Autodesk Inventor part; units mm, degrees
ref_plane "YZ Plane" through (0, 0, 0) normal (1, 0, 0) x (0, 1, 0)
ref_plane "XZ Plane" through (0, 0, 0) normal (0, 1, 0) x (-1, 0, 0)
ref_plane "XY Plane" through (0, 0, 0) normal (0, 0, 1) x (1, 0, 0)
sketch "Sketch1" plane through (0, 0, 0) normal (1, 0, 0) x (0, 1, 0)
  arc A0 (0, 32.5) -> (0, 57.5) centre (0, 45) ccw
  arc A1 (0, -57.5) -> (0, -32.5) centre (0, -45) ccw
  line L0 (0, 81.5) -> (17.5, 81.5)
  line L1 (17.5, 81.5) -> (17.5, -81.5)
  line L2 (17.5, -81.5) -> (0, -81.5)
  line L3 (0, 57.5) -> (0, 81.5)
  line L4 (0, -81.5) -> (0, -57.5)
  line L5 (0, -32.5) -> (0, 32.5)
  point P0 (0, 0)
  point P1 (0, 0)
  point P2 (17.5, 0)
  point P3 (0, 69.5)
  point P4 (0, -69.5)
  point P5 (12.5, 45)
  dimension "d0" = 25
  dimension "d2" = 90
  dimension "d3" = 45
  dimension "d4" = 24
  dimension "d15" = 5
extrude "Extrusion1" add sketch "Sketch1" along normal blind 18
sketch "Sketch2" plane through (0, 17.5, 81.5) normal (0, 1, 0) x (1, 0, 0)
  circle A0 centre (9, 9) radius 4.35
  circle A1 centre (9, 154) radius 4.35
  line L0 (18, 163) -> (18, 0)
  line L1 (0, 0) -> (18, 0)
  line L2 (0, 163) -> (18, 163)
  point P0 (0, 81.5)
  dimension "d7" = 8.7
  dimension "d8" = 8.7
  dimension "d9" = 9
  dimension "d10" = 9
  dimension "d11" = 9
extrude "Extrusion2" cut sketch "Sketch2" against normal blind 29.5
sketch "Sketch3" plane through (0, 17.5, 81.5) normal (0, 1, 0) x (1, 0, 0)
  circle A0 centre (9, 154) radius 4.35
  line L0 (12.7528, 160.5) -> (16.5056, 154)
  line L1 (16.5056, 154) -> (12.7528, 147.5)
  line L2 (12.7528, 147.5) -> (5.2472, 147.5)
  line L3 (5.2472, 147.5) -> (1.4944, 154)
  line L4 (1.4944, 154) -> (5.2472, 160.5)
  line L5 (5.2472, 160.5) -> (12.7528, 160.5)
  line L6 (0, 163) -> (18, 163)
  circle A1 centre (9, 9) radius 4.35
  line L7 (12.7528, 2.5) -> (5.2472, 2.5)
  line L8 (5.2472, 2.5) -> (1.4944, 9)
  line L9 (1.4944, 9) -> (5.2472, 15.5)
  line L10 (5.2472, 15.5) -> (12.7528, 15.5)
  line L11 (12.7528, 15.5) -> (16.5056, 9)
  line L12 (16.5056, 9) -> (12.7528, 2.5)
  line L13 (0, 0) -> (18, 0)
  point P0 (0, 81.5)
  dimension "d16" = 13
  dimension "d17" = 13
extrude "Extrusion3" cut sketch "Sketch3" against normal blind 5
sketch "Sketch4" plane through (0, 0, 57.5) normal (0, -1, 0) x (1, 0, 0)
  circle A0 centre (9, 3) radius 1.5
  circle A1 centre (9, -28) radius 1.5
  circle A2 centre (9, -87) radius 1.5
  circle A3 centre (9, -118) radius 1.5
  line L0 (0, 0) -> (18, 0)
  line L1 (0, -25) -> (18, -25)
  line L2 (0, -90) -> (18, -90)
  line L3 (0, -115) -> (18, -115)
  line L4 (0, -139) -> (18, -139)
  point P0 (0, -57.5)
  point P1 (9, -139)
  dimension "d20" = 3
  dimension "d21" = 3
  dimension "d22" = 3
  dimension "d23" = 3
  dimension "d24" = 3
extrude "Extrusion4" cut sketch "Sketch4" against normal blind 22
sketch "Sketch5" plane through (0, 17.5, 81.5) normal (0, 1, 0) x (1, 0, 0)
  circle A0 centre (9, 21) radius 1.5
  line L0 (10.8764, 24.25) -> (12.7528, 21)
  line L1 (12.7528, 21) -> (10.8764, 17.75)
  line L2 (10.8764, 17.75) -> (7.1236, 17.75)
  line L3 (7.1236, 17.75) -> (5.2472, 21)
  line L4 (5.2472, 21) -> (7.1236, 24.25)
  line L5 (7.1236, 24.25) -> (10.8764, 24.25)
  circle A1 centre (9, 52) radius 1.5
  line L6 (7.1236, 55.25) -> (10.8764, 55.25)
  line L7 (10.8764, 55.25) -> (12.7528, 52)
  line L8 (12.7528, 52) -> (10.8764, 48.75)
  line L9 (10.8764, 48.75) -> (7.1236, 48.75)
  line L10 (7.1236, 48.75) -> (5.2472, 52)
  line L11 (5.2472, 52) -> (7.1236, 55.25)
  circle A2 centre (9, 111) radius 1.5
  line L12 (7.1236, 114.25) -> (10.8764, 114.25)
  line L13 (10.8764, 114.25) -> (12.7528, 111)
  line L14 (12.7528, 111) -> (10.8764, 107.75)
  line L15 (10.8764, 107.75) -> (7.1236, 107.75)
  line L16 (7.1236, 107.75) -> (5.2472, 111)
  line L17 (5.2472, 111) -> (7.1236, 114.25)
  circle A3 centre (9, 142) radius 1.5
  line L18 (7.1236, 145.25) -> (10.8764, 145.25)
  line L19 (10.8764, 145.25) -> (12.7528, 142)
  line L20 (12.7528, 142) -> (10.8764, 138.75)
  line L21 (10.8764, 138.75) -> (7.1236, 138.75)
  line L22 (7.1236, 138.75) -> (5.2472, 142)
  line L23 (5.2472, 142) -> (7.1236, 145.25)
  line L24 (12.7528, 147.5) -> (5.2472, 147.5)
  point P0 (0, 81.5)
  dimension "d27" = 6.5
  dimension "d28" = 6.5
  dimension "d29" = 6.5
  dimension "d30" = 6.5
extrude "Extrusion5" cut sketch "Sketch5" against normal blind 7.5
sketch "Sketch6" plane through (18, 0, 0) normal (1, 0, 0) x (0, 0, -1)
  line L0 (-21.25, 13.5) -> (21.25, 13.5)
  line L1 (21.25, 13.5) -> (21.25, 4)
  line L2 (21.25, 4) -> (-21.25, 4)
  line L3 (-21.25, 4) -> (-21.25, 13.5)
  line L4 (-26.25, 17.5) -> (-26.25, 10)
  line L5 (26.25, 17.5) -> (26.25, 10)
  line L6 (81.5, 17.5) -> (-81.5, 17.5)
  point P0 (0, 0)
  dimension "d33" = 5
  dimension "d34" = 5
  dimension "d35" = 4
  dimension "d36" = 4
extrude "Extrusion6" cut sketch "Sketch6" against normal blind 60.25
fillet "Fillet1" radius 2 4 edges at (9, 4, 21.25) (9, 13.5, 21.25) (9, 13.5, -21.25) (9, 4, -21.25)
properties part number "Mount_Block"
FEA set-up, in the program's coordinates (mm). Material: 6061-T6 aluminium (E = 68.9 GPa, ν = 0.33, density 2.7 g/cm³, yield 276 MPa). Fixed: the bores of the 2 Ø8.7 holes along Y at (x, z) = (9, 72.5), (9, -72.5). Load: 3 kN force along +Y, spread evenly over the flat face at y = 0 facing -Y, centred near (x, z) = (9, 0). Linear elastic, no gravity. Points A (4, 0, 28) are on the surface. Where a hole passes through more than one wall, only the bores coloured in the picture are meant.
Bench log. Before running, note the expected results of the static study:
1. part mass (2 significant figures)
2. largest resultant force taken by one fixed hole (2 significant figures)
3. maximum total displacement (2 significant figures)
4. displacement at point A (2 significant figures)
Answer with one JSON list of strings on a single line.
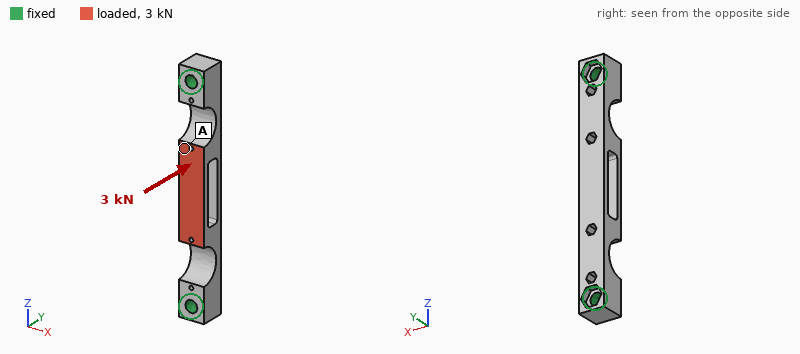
["84 g", "1.6 kN", "0.25 mm", "0.14 mm"]
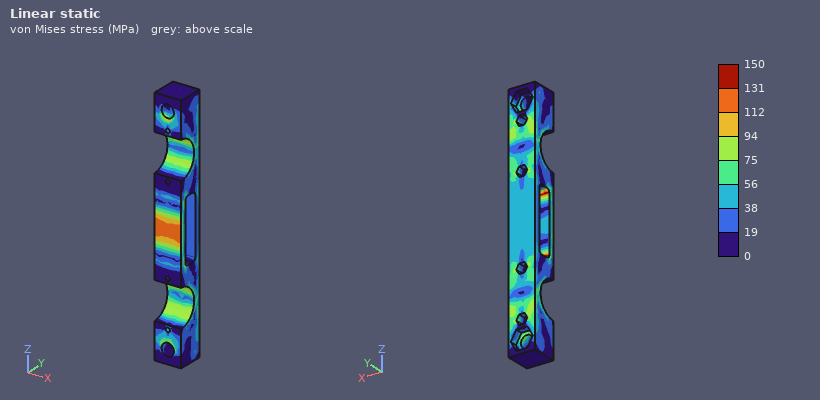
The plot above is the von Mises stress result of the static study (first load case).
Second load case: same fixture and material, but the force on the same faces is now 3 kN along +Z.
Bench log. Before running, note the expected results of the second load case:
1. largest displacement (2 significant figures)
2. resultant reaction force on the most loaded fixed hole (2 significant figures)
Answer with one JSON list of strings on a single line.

["61 µm", "1.6 kN"]
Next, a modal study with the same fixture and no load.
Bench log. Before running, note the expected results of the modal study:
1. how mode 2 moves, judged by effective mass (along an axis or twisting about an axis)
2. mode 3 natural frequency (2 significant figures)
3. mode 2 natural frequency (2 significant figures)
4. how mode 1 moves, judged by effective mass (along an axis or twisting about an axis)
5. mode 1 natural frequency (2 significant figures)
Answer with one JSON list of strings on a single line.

["along Y", "4600 Hz", "3500 Hz", "along X", "3200 Hz"]
